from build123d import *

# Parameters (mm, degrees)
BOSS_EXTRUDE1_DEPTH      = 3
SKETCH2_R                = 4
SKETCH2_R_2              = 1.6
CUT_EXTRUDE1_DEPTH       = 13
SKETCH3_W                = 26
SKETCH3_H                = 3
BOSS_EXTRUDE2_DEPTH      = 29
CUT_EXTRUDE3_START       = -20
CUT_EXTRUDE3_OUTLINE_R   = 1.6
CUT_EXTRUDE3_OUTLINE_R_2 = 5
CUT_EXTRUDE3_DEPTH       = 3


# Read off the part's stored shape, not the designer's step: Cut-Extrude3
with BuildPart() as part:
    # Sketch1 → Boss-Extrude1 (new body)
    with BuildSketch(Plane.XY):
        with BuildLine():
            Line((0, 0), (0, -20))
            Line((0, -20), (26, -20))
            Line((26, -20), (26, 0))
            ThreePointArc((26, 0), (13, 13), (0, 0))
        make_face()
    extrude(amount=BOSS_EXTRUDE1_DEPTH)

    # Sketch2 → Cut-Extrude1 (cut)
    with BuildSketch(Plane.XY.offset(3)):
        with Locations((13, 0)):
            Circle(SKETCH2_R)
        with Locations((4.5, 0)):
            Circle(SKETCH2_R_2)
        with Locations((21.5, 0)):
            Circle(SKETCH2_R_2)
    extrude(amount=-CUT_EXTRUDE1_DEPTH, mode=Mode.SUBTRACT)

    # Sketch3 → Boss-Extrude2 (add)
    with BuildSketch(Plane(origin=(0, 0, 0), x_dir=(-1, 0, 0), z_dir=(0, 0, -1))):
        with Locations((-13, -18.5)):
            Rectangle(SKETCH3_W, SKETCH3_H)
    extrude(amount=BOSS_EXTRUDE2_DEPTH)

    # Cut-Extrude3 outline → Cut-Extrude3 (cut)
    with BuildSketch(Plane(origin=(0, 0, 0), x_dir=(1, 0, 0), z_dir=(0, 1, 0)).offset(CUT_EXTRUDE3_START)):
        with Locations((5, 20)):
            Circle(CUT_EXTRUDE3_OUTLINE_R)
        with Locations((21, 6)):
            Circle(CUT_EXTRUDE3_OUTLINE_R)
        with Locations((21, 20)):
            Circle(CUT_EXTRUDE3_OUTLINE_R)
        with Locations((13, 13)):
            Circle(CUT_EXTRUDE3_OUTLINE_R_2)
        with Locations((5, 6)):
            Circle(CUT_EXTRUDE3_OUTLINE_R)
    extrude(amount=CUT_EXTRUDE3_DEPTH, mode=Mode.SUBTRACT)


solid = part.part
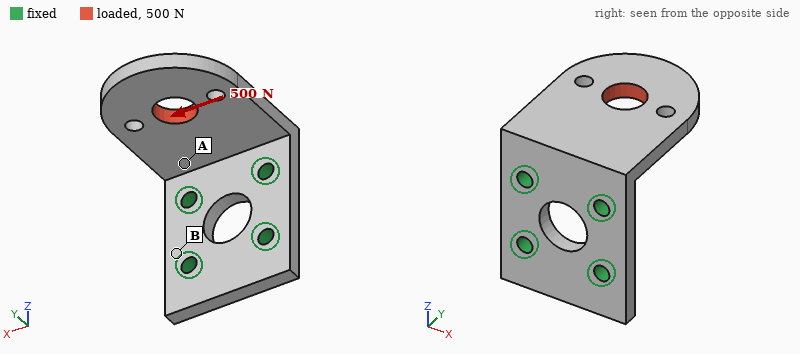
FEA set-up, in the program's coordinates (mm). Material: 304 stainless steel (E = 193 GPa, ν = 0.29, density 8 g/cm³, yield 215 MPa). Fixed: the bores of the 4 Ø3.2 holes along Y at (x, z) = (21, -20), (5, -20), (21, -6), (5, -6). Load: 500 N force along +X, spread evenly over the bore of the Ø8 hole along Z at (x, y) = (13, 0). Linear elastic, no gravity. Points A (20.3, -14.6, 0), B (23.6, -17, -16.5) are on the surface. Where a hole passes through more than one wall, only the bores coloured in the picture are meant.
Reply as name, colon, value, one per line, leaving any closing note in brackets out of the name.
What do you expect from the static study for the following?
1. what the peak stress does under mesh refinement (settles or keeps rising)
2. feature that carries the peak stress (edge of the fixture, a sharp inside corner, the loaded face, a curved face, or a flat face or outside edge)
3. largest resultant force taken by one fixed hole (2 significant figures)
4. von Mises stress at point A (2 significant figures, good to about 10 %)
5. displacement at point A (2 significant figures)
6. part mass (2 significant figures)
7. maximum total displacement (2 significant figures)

what the peak stress does under mesh refinement: keeps rising
feature that carries the peak stress: edge of the fixture
largest resultant force taken by one fixed hole: 600 N
von Mises stress at point A: 54 MPa
displacement at point A: 7.8 µm
part mass: 33 g
maximum total displacement: 34 µm
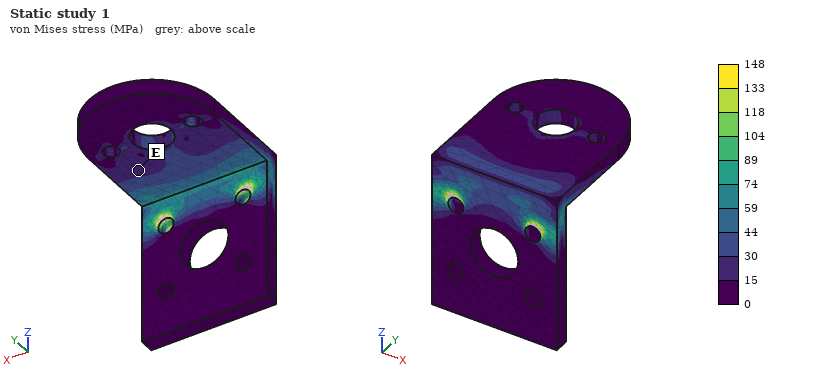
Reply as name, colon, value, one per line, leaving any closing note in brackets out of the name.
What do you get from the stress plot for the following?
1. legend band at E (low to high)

legend band at E: 15 to 30 MPa
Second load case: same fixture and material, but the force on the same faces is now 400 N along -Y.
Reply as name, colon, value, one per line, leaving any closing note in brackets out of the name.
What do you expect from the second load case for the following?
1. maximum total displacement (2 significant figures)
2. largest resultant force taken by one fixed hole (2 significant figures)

maximum total displacement: 30 µm
largest resultant force taken by one fixed hole: 210 N
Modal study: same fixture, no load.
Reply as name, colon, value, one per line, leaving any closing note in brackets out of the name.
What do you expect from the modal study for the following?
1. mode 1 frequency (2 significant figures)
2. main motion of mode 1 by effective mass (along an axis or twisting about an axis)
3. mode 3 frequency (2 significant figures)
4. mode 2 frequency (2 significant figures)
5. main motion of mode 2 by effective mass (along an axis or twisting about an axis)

mode 1 frequency: 2200 Hz
main motion of mode 1 by effective mass: along Z
mode 3 frequency: 8300 Hz
mode 2 frequency: 6000 Hz
main motion of mode 2 by effective mass: along X
